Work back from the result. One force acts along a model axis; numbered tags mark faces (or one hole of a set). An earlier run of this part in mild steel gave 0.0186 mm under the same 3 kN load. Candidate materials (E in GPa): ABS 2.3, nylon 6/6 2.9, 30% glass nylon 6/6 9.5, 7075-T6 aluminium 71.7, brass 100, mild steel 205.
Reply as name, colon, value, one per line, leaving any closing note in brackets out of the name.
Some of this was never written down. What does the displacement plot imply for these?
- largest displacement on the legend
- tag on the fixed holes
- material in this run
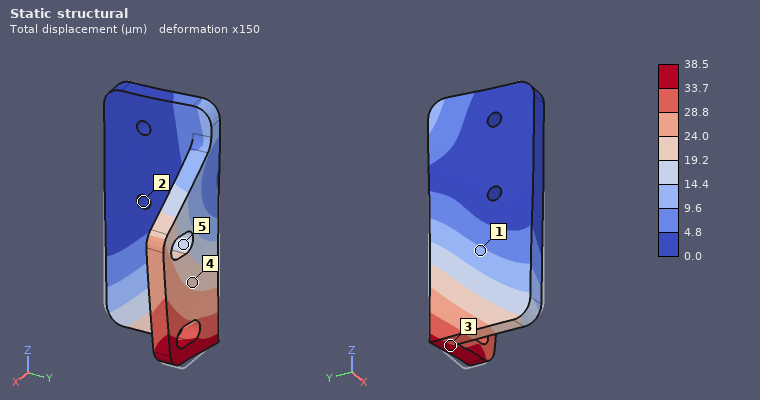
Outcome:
largest displacement on the legend: 38.5 µm
tag on the fixed holes: 2
material in this run: brass
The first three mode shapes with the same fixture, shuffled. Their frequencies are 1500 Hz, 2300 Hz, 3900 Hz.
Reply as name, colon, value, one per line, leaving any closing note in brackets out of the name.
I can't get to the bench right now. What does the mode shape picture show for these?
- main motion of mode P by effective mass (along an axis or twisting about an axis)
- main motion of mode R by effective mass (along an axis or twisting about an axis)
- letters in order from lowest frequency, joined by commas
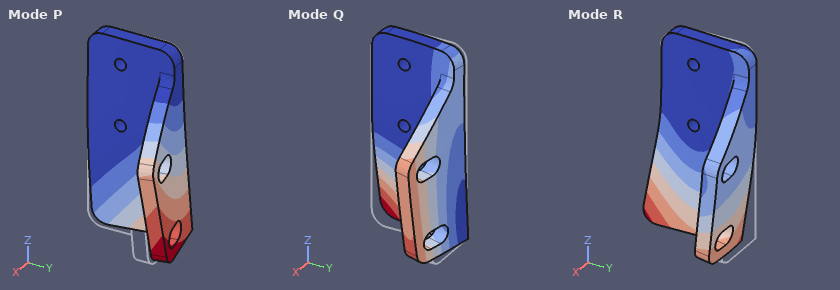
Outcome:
main motion of mode P by effective mass: along X
main motion of mode R by effective mass: along Y
letters in order from lowest frequency, joined by commas: P, Q, R
